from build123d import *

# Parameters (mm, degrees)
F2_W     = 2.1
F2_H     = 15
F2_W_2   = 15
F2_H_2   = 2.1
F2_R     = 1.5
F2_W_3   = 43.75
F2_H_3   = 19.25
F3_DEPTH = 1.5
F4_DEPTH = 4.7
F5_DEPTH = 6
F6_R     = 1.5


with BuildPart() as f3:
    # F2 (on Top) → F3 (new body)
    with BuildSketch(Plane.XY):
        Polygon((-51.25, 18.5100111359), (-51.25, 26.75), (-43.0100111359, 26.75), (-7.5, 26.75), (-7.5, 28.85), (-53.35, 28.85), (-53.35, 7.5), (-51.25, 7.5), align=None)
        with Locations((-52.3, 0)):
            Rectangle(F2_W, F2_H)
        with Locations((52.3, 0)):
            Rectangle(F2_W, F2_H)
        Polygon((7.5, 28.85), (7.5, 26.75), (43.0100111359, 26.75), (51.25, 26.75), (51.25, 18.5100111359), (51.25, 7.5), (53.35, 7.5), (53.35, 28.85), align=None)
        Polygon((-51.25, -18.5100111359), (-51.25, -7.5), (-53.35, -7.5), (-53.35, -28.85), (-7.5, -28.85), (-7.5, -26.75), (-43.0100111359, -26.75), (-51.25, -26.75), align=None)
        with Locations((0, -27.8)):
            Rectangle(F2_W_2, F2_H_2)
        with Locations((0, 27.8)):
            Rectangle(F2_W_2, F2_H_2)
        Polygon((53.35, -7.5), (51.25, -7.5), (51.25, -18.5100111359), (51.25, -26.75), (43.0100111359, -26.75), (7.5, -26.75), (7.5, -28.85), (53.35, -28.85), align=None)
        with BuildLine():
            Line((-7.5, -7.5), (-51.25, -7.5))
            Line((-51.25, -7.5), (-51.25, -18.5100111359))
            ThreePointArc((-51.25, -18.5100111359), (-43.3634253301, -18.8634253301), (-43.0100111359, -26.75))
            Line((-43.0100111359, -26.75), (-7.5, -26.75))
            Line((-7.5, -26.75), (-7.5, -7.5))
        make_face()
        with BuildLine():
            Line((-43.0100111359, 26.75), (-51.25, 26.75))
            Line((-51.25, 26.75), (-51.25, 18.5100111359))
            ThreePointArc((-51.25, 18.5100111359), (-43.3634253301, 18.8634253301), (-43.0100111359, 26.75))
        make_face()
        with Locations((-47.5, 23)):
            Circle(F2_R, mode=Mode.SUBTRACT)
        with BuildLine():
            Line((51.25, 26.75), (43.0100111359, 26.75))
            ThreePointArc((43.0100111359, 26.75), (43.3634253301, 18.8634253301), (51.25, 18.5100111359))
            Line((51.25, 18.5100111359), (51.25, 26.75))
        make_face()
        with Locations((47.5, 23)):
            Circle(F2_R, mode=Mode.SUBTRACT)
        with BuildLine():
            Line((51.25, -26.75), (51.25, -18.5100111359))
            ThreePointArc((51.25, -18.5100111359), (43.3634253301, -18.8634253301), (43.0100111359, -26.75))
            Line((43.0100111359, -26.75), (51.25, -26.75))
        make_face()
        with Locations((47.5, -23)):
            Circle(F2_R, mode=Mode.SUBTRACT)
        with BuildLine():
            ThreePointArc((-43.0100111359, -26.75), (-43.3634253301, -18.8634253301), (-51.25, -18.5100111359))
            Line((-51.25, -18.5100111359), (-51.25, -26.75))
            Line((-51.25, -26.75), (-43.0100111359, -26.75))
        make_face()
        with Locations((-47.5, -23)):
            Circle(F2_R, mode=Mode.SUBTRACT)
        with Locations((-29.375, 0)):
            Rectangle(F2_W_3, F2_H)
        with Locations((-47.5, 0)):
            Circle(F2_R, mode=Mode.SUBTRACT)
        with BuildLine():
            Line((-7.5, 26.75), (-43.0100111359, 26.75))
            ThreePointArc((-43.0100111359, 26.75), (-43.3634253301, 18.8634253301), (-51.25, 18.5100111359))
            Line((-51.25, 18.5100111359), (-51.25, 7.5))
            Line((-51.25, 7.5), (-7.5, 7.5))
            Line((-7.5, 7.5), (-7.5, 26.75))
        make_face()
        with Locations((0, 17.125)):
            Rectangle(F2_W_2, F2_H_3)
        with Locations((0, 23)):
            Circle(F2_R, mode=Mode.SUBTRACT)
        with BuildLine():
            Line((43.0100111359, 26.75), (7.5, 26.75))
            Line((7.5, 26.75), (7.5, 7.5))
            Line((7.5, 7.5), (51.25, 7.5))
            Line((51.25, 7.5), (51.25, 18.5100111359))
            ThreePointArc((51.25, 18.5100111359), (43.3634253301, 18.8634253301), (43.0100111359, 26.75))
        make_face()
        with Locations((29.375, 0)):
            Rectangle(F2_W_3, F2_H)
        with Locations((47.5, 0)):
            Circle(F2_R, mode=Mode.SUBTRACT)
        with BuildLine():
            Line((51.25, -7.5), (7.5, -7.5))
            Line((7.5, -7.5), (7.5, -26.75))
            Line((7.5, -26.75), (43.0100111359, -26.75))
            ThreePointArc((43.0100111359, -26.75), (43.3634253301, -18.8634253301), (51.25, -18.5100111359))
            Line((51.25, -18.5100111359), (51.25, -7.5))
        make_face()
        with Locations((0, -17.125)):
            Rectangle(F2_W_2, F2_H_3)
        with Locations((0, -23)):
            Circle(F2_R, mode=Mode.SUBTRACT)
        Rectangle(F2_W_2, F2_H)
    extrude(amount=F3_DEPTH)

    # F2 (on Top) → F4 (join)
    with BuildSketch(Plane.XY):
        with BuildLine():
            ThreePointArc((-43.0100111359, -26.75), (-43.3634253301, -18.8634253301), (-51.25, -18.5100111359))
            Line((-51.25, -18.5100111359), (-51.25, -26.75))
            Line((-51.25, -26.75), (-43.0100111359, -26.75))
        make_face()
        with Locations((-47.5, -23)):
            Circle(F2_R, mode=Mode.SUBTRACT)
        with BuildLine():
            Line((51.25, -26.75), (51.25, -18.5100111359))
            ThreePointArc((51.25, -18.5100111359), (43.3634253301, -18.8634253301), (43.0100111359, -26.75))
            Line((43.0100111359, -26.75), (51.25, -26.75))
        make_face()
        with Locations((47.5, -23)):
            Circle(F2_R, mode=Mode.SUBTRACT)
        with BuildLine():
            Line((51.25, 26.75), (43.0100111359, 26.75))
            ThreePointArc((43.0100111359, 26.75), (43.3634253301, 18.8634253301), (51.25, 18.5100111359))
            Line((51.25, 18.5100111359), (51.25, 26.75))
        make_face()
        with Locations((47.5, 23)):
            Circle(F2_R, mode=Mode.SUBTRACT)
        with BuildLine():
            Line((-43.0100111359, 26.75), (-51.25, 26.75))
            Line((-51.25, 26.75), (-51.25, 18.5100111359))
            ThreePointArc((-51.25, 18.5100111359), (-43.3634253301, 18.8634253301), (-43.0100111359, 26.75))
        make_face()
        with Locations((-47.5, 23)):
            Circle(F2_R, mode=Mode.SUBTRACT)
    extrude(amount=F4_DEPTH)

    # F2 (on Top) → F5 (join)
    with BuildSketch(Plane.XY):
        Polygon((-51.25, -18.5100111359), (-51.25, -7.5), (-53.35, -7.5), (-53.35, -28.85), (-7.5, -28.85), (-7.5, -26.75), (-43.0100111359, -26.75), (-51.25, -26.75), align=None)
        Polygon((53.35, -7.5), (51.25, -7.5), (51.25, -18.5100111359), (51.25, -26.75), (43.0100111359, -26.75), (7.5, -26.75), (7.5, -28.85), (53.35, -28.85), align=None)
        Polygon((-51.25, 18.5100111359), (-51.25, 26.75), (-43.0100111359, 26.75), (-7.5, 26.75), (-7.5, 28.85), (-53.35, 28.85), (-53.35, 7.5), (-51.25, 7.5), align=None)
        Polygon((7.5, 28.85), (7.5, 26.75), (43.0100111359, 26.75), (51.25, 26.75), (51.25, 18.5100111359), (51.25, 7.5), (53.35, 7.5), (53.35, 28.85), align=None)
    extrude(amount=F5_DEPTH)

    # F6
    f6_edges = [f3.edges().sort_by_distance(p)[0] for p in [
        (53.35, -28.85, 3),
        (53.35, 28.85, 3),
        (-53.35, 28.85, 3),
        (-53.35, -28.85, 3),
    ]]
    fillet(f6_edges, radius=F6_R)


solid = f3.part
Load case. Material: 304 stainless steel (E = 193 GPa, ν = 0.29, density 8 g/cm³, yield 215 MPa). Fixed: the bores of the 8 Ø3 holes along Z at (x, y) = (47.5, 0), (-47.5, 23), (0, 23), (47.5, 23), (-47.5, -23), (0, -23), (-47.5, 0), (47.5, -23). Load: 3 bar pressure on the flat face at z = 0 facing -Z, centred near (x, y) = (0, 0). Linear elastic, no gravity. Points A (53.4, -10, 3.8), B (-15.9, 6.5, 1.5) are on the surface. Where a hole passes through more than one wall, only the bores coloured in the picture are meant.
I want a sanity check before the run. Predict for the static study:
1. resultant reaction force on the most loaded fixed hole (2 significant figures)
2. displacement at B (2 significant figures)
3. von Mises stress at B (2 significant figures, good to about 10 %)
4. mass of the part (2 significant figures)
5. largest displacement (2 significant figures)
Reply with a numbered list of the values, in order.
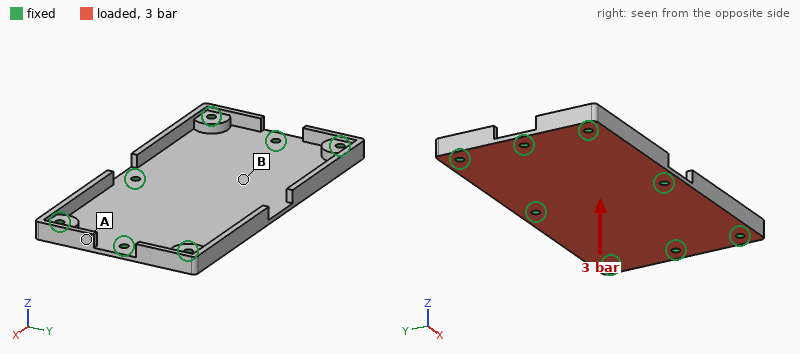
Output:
1. 370 N
2. 88 µm
3. 59 MPa
4. 100 g
5. 97 µm
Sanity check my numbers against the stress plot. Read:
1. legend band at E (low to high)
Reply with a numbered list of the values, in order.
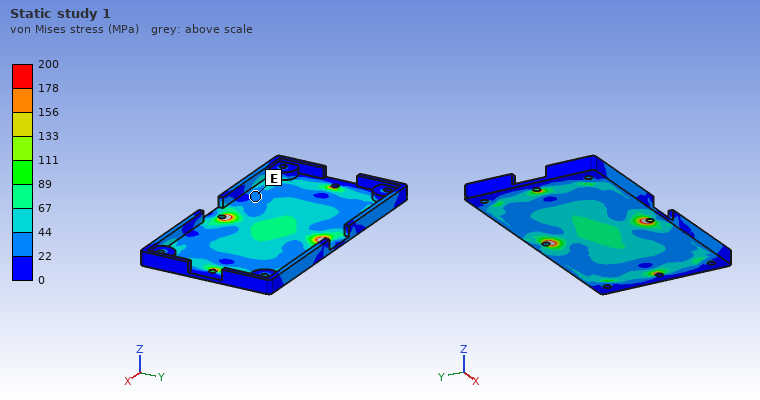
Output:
1. 22 to 44 MPa
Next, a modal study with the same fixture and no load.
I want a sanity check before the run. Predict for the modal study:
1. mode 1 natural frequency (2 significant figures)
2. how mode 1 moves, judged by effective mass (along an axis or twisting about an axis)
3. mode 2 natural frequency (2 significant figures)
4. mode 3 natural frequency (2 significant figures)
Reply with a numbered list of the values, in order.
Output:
1. 3100 Hz
2. along Z
3. 3600 Hz
4. 6200 Hz
